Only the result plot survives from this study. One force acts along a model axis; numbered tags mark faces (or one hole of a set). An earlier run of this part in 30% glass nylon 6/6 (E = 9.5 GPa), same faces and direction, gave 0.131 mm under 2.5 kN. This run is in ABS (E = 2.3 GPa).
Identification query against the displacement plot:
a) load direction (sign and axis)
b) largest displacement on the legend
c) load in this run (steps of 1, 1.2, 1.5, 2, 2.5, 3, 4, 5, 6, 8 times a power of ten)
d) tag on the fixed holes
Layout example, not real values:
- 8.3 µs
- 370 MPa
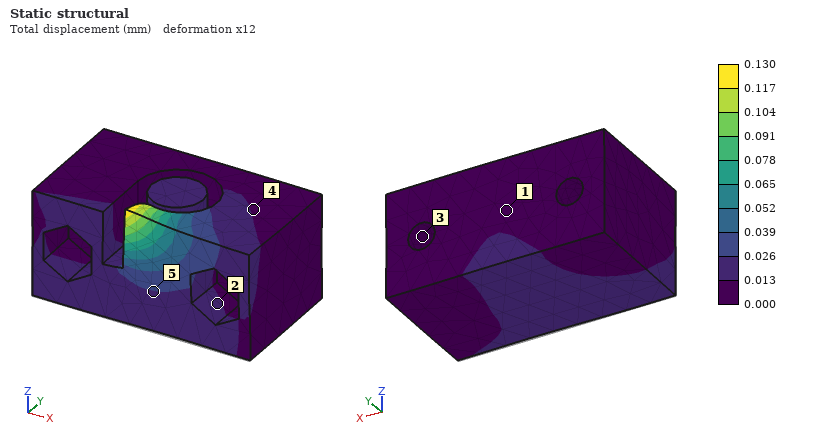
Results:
- +Y
- 0.130 mm
- 600 N
- 3
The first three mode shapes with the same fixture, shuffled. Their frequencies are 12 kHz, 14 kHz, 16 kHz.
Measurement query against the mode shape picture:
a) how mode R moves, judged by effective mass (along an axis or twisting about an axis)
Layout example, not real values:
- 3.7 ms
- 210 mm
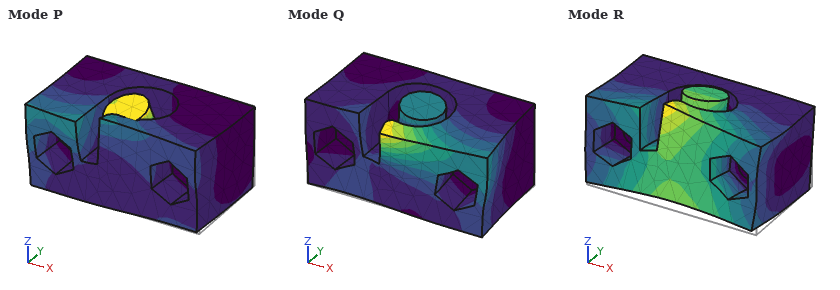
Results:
- along Z
